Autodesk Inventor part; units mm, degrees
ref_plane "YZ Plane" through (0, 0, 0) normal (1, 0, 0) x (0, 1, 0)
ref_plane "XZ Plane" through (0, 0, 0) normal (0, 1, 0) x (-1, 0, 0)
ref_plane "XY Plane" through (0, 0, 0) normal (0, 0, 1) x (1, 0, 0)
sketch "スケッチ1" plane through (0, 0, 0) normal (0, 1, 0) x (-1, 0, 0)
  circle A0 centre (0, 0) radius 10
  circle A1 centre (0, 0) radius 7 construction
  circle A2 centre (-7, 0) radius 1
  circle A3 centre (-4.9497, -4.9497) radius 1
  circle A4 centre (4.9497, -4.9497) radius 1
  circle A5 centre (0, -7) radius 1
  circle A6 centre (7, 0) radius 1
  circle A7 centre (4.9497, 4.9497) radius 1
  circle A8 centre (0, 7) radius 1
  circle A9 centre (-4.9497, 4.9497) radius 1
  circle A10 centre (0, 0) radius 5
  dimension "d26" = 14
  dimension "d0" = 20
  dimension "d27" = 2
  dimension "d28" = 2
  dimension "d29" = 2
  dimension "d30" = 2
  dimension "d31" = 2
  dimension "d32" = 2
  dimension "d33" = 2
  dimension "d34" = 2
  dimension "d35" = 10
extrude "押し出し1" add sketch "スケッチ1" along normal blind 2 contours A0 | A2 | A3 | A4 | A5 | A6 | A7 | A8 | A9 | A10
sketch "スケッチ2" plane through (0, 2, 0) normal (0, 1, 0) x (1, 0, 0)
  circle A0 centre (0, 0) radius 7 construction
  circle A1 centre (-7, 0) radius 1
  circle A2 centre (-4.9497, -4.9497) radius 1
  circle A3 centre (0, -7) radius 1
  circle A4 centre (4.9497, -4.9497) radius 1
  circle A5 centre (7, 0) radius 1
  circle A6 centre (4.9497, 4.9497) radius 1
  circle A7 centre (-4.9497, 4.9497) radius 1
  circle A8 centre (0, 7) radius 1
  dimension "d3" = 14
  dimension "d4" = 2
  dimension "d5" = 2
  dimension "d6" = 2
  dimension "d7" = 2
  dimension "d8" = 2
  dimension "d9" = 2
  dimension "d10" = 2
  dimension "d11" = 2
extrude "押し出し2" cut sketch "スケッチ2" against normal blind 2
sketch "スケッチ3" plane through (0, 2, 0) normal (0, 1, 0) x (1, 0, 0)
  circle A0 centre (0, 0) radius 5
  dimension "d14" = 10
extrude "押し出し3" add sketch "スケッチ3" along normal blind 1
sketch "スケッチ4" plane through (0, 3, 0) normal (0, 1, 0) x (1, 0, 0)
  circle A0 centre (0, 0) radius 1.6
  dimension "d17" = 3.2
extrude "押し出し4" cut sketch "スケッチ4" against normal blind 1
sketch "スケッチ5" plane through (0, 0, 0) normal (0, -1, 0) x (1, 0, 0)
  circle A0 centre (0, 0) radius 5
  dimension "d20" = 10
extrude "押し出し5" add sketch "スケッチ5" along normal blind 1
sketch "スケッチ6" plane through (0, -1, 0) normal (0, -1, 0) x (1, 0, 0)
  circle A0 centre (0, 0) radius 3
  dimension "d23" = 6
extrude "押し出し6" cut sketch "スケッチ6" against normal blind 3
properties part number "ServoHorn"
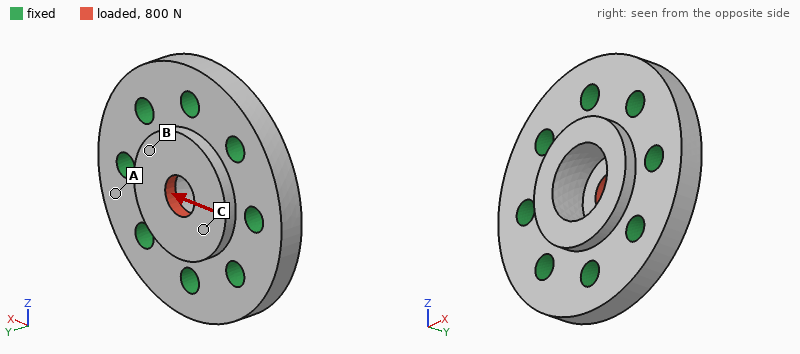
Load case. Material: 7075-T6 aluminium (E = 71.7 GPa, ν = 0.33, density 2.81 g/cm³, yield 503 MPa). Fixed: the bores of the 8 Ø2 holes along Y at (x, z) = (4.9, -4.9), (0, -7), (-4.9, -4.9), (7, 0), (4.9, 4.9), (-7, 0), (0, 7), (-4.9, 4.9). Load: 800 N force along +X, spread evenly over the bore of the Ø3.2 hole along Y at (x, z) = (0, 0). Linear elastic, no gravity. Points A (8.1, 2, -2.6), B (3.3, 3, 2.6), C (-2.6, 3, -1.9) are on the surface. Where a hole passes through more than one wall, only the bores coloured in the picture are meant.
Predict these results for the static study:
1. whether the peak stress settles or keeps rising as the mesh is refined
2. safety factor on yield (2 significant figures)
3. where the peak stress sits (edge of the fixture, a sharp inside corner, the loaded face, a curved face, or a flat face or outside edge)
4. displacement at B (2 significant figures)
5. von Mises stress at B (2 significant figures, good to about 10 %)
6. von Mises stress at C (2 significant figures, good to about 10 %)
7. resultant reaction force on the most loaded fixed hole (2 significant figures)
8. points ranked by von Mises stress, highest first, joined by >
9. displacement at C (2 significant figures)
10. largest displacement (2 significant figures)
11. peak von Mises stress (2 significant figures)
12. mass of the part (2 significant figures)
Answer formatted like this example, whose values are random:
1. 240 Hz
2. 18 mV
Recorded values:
1. settles
2. 3.4
3. the loaded face
4. 2.0 µm
5. 29 MPa
6. 49 MPa
7. 170 N
8. C > B > A
9. 2.7 µm
10. 5.1 µm
11. 150 MPa
12. 1.8 g
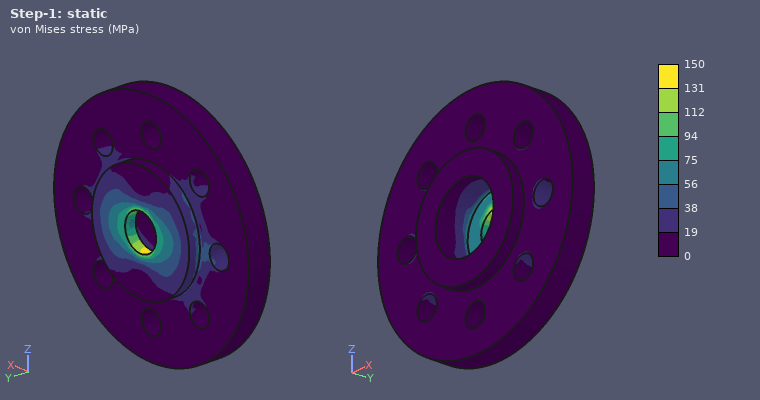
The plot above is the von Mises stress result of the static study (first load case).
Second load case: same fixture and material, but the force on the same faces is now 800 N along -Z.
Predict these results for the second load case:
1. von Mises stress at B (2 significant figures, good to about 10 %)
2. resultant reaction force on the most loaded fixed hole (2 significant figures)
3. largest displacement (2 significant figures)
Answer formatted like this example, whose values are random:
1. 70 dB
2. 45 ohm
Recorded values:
1. 22 MPa
2. 170 N
3. 5.0 µm
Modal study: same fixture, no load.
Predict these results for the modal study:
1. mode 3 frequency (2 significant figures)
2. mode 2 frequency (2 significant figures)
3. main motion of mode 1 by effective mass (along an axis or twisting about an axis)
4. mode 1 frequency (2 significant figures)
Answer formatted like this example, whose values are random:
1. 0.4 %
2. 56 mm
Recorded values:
1. 150 kHz
2. 150 kHz
3. along Y
4. 120 kHz
